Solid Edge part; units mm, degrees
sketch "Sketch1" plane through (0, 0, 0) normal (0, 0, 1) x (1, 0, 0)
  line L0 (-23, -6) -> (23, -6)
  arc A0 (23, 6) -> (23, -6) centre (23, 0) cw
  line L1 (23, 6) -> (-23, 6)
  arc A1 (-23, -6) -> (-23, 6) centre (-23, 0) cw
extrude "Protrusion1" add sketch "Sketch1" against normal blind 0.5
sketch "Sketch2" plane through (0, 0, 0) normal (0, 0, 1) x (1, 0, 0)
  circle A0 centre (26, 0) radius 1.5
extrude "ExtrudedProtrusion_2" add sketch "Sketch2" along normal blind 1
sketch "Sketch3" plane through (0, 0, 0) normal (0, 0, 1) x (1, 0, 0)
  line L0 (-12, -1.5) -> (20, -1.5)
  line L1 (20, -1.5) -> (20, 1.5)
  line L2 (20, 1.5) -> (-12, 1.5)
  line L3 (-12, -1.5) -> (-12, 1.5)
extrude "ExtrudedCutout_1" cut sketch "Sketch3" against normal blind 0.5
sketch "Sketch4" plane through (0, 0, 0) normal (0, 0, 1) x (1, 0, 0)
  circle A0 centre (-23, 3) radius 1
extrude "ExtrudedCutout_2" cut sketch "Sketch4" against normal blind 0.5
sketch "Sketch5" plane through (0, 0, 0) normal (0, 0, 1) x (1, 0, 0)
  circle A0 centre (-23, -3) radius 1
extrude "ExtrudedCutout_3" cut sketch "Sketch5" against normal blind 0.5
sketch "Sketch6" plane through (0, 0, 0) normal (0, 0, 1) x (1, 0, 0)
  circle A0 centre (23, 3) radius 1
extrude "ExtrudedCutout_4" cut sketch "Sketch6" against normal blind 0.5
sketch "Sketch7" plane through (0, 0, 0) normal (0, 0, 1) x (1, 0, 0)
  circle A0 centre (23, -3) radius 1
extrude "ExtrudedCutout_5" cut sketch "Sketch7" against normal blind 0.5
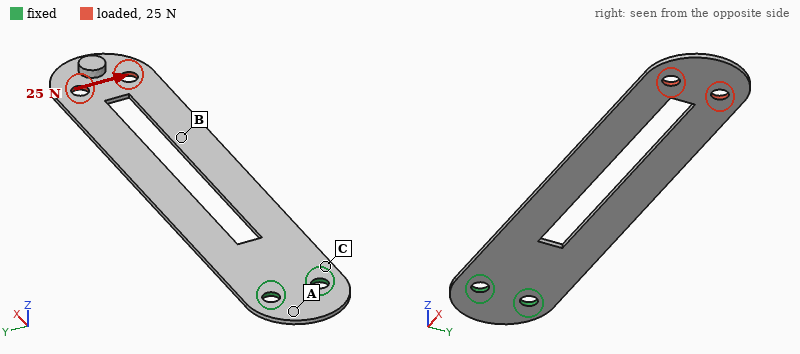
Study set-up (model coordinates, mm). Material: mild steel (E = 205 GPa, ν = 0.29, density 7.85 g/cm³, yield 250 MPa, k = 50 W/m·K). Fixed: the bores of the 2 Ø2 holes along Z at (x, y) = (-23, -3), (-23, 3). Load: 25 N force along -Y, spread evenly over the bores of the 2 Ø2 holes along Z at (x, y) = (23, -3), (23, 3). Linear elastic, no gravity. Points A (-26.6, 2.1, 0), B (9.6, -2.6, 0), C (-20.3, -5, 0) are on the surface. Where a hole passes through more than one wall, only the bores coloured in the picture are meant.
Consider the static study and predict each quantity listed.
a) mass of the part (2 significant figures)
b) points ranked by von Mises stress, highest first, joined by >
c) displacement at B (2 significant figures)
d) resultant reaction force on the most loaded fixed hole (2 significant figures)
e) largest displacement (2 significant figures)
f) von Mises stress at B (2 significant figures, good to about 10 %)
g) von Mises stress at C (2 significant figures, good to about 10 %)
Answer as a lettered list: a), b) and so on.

a) 2.2 g
b) C > B > A
c) 0.078 mm
d) 160 N
e) 0.13 mm
f) 39 MPa
g) 69 MPa
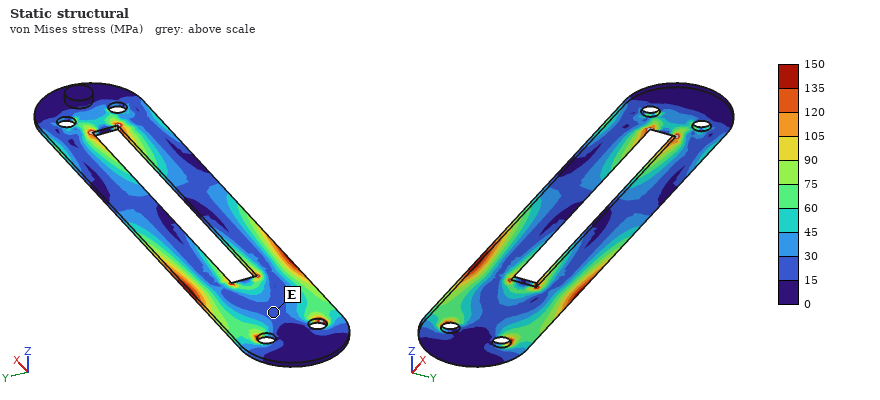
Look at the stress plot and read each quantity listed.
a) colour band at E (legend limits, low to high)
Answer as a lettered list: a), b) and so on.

a) 15 to 30 MPa
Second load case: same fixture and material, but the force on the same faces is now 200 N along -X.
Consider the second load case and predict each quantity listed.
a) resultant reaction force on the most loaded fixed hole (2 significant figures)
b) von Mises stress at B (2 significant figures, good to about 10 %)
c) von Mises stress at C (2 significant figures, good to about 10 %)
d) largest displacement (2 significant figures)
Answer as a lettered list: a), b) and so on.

a) 100 N
b) 47 MPa
c) 31 MPa
d) 10 µm
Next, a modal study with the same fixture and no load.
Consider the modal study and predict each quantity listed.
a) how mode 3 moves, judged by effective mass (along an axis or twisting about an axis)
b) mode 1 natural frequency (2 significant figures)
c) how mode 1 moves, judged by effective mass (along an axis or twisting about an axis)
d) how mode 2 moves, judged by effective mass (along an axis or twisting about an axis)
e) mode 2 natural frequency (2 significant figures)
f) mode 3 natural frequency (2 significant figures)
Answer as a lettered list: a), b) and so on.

a) twisting about X
b) 160 Hz
c) along Z
d) along Z
e) 1000 Hz
f) 1100 Hz
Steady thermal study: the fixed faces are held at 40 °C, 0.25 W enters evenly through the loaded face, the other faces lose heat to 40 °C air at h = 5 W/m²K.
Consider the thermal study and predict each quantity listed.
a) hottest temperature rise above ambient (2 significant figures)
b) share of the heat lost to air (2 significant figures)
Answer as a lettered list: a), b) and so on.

a) 35 K
b) 38 %
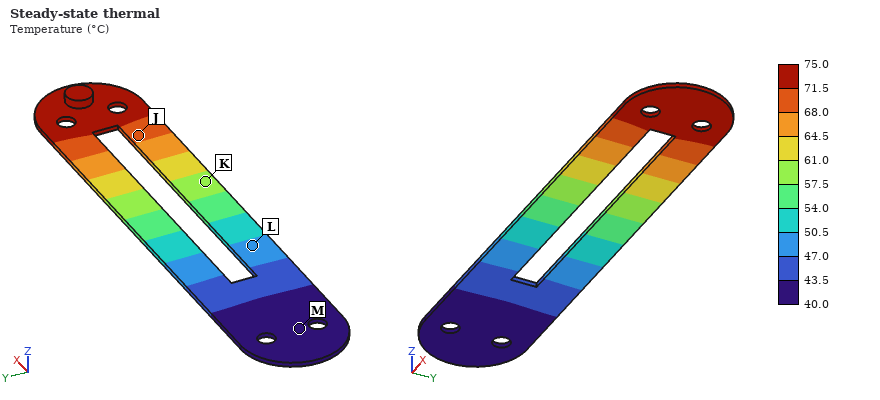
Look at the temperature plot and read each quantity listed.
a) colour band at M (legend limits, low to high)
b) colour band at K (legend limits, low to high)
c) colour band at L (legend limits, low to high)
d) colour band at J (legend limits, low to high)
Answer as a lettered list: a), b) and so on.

a) 40.0 to 43.5 °C
b) 57.5 to 61.0 °C
c) 47.0 to 50.5 °C
d) 68.0 to 71.5 °C
